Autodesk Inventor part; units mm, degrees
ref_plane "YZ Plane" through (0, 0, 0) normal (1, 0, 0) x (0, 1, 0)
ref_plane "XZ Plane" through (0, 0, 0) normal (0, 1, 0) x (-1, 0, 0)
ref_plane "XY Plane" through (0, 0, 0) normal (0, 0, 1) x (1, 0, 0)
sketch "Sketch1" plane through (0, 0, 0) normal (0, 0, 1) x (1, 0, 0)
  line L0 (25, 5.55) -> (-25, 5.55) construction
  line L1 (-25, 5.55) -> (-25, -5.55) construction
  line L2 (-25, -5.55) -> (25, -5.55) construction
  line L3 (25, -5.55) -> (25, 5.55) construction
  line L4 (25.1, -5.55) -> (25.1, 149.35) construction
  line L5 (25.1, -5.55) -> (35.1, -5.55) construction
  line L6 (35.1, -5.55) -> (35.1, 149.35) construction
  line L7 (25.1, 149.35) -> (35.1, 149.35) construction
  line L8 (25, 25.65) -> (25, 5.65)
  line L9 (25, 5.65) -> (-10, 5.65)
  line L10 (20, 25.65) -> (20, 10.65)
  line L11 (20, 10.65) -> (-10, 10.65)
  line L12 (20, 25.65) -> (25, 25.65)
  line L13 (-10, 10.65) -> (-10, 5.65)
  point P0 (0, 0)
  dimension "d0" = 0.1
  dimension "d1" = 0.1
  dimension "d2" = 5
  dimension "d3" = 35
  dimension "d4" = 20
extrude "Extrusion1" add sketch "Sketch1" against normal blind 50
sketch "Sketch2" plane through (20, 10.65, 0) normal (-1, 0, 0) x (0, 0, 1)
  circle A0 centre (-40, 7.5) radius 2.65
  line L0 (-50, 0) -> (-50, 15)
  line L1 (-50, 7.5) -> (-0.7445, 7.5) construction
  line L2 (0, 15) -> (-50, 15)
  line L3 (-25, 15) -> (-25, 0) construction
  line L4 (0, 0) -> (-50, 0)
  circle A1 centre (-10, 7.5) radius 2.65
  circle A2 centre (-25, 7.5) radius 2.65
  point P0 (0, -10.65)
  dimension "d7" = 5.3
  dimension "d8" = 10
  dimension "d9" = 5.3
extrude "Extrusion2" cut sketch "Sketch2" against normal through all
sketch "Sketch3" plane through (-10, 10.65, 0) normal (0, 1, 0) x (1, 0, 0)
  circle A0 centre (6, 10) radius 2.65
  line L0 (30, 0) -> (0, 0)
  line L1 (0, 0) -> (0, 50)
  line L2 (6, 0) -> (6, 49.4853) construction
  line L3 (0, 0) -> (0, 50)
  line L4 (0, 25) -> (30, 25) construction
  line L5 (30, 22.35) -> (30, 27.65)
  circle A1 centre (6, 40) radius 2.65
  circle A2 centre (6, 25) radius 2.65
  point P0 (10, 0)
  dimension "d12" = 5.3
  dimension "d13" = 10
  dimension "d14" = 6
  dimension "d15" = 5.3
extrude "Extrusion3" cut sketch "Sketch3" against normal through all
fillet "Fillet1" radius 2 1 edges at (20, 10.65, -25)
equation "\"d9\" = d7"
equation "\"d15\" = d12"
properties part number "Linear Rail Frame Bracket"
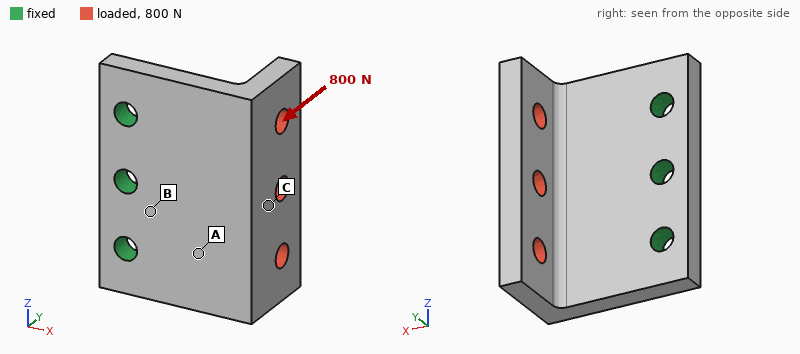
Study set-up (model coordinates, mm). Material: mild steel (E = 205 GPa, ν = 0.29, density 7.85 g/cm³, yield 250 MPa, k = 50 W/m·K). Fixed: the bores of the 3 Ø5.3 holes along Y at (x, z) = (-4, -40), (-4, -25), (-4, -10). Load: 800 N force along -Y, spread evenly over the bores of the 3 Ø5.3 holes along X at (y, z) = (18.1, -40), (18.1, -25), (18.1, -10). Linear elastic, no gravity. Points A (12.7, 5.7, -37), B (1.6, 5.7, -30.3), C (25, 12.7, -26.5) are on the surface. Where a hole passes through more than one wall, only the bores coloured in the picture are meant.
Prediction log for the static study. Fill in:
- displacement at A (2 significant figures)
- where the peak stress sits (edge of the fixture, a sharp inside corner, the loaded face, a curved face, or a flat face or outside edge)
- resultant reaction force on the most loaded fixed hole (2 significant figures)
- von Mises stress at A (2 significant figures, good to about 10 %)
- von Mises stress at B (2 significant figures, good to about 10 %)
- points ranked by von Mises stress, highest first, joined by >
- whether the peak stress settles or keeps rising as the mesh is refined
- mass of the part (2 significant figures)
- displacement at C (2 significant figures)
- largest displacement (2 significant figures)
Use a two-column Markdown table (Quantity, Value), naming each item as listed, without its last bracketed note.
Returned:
| Quantity | Value |
|---|---|
| displacement at A | 19 µm |
| where the peak stress sits | edge of the fixture |
| resultant reaction force on the most loaded fixed hole | 280 N |
| von Mises stress at A | 34 MPa |
| von Mises stress at B | 67 MPa |
| points ranked by von Mises stress, highest first, joined by > | B > A > C |
| whether the peak stress settles or keeps rising as the mesh is refined | keeps rising |
| mass of the part | 93 g |
| displacement at C | 48 µm |
| largest displacement | 62 µm |
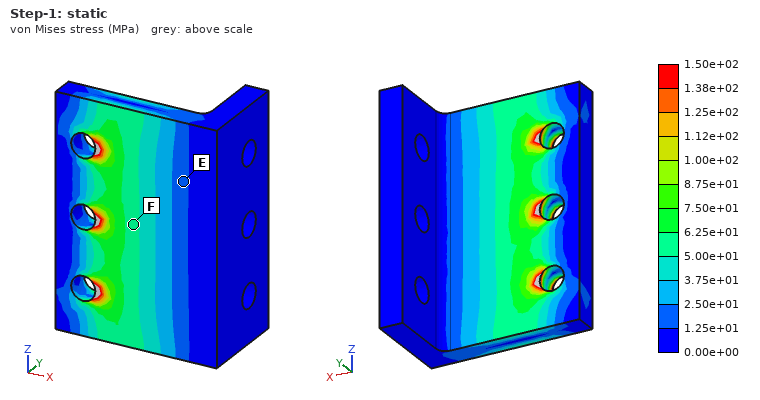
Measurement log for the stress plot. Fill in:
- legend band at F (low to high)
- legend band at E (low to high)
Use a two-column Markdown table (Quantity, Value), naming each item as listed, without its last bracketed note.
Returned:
| Quantity | Value |
|---|---|
| legend band at F | 5.00e+01 to 6.25e+01 MPa |
| legend band at E | 1.25e+01 to 2.50e+01 MPa |
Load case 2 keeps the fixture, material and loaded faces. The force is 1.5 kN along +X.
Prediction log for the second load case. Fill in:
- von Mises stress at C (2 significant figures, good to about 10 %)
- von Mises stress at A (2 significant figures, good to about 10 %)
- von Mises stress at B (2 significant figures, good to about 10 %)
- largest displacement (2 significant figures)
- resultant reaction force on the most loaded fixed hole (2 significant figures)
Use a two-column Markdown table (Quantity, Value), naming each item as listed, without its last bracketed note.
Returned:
| Quantity | Value |
|---|---|
| von Mises stress at C | 33 MPa |
| von Mises stress at A | 58 MPa |
| von Mises stress at B | 56 MPa |
| largest displacement | 83 µm |
| resultant reaction force on the most loaded fixed hole | 510 N |
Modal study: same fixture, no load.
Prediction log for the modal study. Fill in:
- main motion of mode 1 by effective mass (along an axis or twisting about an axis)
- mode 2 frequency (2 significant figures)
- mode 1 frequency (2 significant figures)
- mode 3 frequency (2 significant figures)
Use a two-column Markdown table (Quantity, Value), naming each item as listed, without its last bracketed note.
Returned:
| Quantity | Value |
|---|---|
| main motion of mode 1 by effective mass | along Y |
| mode 2 frequency | 5000 Hz |
| mode 1 frequency | 3000 Hz |
| mode 3 frequency | 10 kHz |
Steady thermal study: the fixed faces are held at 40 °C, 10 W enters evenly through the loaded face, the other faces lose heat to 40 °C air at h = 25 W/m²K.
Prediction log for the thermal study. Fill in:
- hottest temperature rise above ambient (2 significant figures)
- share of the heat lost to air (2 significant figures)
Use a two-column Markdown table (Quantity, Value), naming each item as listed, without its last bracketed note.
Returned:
| Quantity | Value |
|---|---|
| hottest temperature rise above ambient | 26 K |
| share of the heat lost to air | 17 % |
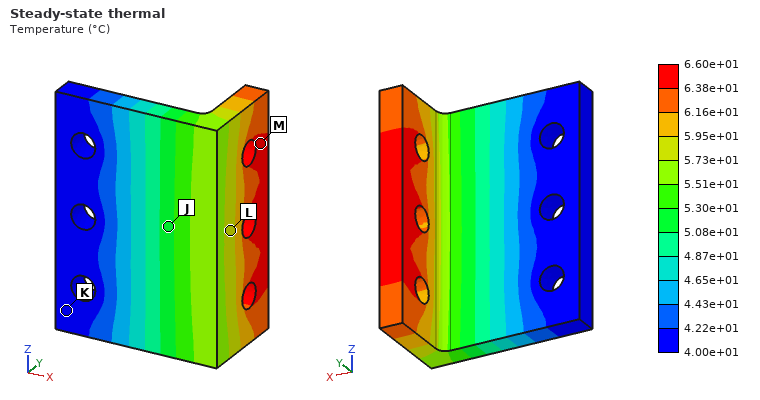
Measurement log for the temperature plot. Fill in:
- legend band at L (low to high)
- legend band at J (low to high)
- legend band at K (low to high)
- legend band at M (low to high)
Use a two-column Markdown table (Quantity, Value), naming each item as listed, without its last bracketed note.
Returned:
| Quantity | Value |
|---|---|
| legend band at L | 5.73e+01 to 5.95e+01 °C |
| legend band at J | 5.08e+01 to 5.30e+01 °C |
| legend band at K | 4.00e+01 to 4.22e+01 °C |
| legend band at M | 6.38e+01 to 6.60e+01 °C |
